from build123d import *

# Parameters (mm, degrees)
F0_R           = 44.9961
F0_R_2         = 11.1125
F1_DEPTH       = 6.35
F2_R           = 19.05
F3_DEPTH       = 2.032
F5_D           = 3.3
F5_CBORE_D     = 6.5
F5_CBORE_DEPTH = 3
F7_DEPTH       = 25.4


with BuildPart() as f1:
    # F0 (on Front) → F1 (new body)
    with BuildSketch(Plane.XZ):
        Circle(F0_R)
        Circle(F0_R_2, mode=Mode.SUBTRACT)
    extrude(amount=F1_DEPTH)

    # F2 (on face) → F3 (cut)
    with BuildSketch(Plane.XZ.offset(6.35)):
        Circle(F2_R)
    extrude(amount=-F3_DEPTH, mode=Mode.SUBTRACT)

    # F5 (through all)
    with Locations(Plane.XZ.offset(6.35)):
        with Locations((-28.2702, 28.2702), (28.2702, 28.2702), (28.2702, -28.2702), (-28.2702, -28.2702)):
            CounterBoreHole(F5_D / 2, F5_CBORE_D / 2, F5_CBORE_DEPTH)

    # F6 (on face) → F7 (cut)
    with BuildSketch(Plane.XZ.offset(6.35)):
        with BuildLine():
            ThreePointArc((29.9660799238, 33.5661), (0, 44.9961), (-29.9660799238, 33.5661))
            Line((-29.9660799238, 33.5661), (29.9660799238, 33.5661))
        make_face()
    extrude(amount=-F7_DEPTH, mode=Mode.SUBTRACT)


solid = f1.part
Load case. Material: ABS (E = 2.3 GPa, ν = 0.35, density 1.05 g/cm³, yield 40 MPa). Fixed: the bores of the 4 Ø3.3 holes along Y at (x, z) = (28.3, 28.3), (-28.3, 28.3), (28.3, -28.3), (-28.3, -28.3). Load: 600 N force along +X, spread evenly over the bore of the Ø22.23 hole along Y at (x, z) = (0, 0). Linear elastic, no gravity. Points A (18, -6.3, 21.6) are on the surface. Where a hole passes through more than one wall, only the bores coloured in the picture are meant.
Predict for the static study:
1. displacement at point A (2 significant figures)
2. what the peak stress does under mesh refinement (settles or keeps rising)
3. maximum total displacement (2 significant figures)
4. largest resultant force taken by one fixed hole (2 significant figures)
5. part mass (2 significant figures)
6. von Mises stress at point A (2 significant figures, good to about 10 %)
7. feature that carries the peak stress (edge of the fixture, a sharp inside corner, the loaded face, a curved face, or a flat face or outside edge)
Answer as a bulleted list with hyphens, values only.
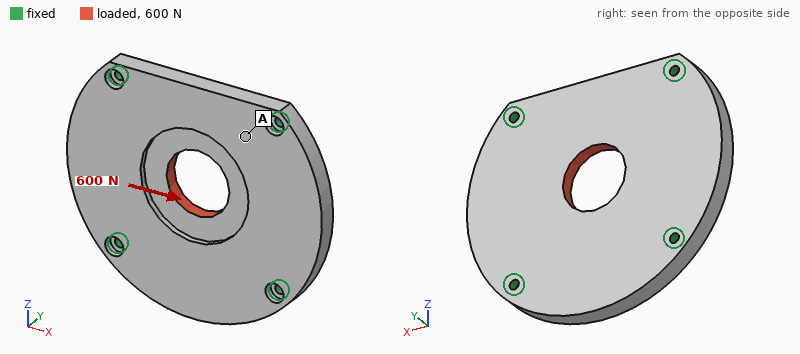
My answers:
- 17 µm
- keeps rising
- 36 µm
- 150 N
- 35 g
- 0.87 MPa
- edge of the fixture
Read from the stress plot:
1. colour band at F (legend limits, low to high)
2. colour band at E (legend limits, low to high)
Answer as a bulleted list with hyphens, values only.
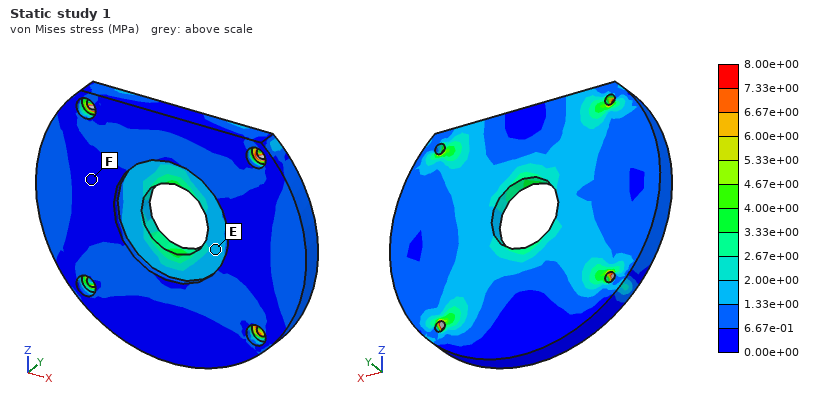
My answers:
- 0.00e+00 to 6.67e-01 MPa
- 1.33e+00 to 2.00e+00 MPa
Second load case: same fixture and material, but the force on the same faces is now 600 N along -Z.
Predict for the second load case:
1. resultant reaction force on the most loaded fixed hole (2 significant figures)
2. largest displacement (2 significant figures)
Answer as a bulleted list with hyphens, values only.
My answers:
- 160 N
- 43 µm
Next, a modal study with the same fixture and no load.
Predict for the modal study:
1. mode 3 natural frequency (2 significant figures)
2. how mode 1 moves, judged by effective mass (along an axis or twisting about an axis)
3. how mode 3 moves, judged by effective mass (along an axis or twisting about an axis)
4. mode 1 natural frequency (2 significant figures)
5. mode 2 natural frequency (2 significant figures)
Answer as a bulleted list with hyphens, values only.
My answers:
- 1900 Hz
- along Y
- twisting about Z
- 1600 Hz
- 1700 Hz
